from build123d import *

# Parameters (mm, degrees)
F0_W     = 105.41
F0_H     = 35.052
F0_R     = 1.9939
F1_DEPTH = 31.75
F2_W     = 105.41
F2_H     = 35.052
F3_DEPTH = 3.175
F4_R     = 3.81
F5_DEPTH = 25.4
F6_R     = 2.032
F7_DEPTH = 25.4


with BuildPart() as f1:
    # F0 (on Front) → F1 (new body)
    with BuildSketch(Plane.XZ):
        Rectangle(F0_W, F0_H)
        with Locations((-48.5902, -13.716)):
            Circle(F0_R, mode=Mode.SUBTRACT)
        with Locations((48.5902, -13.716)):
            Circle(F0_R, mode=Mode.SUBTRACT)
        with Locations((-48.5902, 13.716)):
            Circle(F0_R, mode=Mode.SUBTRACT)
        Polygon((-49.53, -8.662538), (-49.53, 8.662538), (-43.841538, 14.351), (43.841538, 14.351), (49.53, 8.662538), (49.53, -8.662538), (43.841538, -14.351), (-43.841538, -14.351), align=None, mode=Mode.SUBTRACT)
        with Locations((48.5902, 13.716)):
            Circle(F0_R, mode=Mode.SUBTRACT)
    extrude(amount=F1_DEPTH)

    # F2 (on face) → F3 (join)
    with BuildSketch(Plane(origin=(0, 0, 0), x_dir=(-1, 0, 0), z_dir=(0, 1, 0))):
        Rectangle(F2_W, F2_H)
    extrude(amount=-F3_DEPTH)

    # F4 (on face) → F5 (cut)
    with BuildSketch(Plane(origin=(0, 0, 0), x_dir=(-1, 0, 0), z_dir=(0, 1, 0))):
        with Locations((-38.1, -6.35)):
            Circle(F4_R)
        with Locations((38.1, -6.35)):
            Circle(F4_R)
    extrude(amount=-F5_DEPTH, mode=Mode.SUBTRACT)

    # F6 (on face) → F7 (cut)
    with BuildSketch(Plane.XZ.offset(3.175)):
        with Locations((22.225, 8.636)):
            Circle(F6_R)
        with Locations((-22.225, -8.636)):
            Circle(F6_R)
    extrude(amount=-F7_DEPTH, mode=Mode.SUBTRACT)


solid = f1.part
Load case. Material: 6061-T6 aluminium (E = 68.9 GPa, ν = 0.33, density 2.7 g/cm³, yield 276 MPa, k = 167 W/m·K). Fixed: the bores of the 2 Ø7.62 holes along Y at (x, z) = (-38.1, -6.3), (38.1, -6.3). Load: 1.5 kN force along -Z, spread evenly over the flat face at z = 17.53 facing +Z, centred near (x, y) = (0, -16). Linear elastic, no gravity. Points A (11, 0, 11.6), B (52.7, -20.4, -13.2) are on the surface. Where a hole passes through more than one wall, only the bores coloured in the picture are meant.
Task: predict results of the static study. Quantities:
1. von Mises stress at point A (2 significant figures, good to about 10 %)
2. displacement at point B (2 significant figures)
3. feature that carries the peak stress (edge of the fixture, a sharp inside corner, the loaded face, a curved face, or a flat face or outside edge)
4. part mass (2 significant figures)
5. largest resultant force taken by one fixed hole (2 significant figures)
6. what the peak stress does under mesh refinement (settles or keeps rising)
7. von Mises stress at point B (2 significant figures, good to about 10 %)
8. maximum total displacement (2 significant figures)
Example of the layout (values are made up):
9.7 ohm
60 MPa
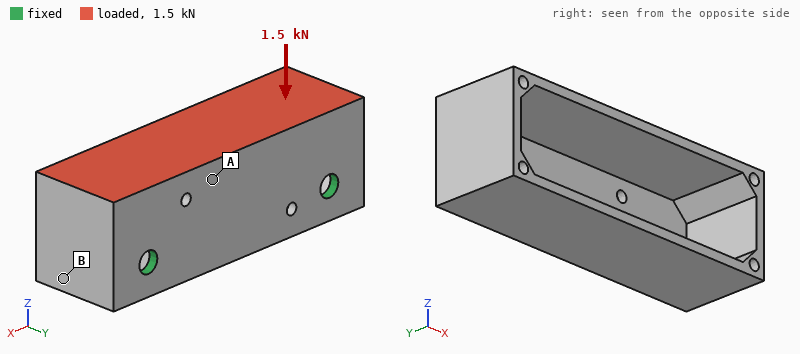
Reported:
46 MPa
0.080 mm
edge of the fixture
98 g
750 N
keeps rising
17 MPa
0.39 mm
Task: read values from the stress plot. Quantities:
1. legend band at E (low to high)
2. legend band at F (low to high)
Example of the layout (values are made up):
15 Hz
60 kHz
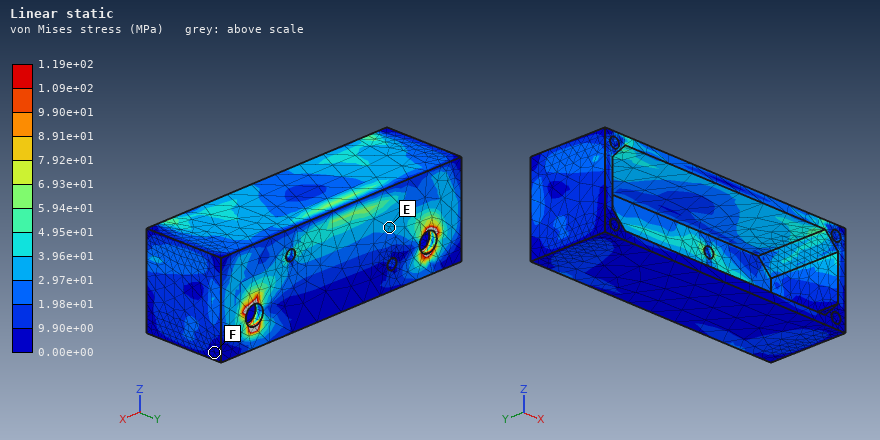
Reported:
2.97e+01 to 3.96e+01 MPa
0.00e+00 to 9.90e+00 MPa
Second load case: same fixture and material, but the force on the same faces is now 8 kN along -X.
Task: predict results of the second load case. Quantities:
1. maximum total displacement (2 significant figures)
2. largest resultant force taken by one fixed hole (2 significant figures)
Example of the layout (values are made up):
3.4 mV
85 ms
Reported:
0.39 mm
4.8 kN
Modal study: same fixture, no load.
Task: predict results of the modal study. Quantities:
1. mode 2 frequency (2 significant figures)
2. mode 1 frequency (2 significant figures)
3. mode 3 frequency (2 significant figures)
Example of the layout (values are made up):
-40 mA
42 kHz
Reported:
2400 Hz
1700 Hz
3100 Hz
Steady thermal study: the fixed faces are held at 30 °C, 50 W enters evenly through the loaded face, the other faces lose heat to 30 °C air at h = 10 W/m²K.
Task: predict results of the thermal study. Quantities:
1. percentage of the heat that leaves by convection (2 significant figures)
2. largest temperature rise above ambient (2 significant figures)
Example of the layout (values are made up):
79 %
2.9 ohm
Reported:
5.8 %
32 K
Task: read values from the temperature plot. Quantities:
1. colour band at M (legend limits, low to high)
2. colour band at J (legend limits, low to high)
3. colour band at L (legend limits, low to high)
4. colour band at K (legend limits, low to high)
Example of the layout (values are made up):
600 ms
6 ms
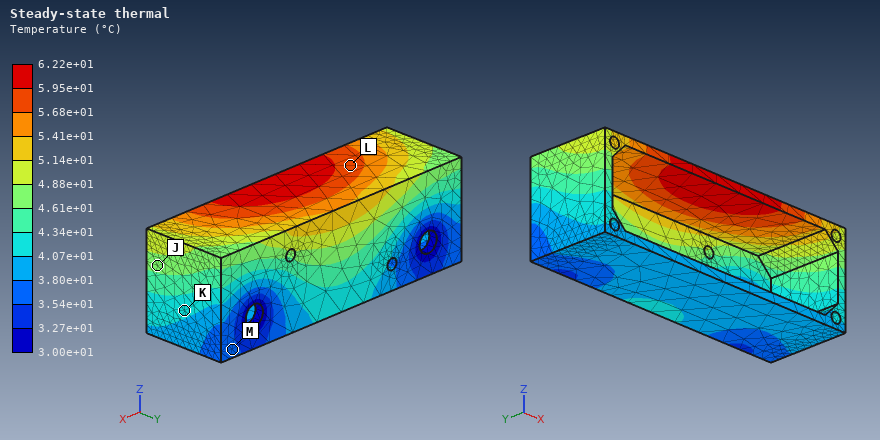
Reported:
3.54e+01 to 3.80e+01 °C
4.61e+01 to 4.88e+01 °C
5.68e+01 to 5.95e+01 °C
4.07e+01 to 4.34e+01 °C
